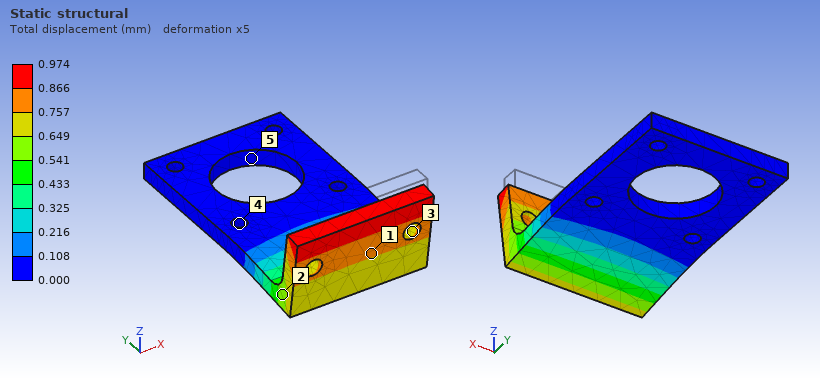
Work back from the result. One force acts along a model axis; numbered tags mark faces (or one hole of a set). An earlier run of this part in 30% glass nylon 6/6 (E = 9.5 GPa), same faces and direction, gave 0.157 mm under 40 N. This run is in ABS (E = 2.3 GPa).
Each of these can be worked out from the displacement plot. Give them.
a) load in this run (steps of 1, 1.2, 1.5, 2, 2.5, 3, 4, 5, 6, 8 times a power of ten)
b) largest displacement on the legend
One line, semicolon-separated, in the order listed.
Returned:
60 N; 0.974 mm
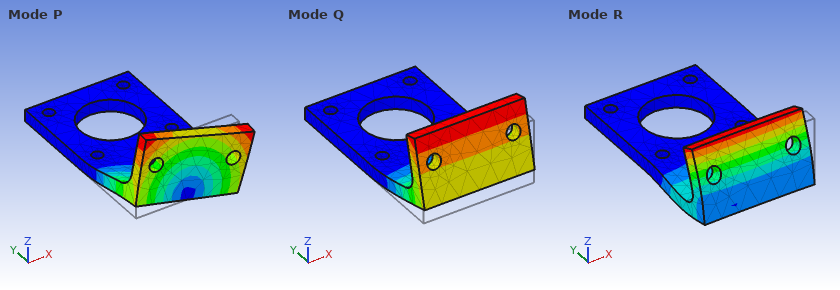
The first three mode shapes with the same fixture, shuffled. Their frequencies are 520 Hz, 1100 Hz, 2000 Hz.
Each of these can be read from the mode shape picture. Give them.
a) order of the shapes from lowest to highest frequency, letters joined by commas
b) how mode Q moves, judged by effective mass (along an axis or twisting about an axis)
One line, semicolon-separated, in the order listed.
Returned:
Q, P, R; along Z
